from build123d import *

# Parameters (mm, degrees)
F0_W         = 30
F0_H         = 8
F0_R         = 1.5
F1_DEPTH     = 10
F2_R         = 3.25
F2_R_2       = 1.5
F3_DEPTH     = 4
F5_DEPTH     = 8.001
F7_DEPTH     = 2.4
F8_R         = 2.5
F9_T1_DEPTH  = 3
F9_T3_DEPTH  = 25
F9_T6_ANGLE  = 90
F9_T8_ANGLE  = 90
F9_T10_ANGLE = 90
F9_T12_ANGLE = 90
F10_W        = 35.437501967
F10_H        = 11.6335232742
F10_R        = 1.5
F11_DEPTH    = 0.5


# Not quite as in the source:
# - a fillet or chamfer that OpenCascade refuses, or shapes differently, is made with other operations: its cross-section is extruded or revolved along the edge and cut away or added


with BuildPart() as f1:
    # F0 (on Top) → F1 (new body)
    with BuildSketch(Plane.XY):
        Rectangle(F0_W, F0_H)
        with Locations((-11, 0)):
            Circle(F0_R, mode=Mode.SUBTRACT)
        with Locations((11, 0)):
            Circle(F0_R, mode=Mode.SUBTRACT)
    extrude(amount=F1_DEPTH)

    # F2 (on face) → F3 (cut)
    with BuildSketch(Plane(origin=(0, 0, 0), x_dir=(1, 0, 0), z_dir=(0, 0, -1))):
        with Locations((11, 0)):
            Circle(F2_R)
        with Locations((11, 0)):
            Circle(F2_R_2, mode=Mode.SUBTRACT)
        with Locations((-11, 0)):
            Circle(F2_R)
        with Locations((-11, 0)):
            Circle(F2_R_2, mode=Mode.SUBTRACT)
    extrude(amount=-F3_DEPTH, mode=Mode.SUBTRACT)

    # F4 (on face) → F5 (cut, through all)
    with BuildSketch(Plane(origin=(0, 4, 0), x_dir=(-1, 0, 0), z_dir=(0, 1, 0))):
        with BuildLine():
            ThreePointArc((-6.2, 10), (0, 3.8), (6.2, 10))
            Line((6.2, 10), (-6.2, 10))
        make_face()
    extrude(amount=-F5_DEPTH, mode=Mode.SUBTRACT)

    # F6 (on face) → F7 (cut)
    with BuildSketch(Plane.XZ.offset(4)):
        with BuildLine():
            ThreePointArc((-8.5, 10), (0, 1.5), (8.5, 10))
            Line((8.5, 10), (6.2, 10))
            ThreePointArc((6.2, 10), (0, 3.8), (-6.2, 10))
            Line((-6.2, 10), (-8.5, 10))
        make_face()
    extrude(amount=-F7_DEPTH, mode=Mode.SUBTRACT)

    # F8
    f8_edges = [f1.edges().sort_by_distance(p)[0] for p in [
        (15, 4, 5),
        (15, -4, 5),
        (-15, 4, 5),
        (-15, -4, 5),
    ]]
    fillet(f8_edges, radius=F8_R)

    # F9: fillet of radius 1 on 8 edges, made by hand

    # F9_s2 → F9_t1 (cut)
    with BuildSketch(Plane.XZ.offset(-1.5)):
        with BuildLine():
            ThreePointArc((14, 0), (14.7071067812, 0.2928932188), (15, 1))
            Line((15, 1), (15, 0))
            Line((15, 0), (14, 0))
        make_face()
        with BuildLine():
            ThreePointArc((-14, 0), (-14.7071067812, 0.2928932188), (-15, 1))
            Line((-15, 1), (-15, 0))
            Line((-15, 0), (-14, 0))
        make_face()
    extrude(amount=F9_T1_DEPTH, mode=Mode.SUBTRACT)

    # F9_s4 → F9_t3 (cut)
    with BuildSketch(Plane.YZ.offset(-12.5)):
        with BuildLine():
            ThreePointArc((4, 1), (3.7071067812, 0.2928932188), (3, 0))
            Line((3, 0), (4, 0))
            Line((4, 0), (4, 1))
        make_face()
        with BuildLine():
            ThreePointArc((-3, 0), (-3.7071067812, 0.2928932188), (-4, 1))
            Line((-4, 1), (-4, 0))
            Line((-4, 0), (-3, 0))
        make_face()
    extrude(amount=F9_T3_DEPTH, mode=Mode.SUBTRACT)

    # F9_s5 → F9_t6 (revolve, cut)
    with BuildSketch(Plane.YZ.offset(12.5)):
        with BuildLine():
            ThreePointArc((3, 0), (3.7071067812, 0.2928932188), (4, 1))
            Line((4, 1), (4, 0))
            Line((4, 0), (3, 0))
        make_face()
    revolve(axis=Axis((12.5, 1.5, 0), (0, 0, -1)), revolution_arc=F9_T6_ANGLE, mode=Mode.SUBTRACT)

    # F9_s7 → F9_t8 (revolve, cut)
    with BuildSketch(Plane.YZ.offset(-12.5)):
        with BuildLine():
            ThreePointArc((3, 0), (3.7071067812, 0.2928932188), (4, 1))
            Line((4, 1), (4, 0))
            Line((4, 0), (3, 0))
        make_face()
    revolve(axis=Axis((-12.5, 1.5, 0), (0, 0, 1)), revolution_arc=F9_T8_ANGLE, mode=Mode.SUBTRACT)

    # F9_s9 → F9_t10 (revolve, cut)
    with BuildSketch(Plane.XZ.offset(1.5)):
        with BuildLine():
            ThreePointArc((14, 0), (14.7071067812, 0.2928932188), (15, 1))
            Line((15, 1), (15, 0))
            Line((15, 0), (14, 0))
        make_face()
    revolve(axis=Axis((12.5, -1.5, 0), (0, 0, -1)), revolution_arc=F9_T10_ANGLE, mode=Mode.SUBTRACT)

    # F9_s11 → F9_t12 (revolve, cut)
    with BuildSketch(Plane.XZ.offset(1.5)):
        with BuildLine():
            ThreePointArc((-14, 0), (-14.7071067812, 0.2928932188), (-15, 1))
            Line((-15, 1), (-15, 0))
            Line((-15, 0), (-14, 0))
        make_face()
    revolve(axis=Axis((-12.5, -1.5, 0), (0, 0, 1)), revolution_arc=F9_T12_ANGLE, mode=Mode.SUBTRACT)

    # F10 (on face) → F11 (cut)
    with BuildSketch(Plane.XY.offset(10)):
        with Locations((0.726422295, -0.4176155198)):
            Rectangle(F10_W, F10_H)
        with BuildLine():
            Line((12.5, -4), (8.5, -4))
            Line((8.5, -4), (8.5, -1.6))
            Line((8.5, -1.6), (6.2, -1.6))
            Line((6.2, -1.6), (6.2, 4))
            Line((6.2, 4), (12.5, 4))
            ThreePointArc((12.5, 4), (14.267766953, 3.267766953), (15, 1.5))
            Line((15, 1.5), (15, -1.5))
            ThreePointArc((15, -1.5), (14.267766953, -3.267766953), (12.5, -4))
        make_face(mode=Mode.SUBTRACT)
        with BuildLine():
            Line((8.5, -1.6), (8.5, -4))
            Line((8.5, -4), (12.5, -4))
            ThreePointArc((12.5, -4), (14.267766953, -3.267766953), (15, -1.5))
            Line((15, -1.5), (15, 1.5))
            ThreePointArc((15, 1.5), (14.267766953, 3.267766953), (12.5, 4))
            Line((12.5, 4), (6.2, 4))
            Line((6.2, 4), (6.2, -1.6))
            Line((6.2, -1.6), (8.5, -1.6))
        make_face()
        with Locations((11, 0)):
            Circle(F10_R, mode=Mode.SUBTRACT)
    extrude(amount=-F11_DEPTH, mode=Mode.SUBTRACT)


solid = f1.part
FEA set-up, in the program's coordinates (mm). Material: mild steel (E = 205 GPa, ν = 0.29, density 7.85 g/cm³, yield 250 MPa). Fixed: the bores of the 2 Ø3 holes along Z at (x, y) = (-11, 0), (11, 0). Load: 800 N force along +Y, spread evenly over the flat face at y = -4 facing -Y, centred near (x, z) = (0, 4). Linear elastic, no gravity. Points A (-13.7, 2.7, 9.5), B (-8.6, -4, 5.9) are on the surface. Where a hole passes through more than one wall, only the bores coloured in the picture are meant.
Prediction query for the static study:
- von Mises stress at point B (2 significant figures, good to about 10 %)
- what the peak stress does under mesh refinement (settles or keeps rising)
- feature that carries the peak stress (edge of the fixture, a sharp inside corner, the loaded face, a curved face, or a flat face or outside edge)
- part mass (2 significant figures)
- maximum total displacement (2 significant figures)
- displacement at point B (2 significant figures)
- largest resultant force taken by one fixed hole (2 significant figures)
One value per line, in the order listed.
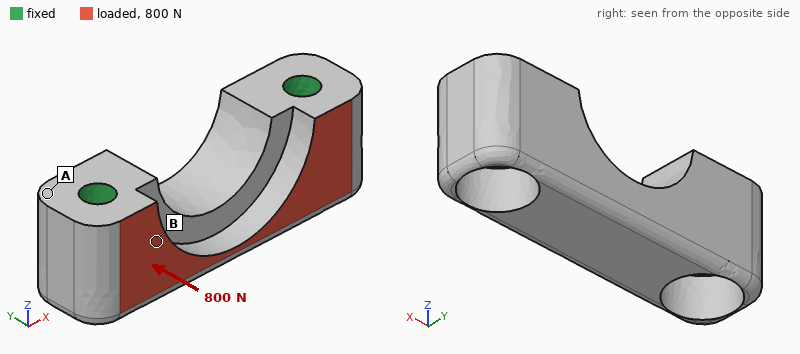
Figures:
22 MPa
keeps rising
edge of the fixture
10 g
1.8 µm
0.57 µm
400 N
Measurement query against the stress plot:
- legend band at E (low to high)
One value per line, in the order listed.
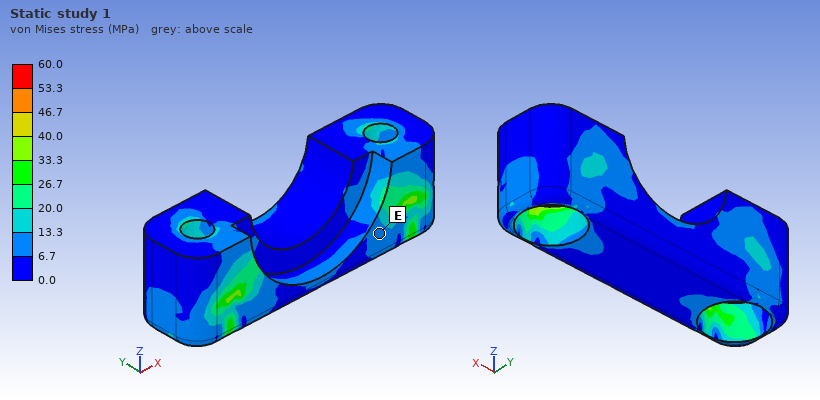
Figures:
6.7 to 13.3 MPa
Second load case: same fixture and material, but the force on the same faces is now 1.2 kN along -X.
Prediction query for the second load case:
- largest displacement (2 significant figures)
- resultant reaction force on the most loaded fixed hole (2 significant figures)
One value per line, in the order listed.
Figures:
1.8 µm
620 N
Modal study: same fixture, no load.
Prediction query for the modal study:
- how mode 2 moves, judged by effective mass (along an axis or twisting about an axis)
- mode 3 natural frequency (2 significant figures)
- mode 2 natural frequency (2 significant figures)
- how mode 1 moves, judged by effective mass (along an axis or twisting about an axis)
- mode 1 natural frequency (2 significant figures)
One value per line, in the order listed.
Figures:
along Z
64 kHz
61 kHz
along Y
38 kHz
